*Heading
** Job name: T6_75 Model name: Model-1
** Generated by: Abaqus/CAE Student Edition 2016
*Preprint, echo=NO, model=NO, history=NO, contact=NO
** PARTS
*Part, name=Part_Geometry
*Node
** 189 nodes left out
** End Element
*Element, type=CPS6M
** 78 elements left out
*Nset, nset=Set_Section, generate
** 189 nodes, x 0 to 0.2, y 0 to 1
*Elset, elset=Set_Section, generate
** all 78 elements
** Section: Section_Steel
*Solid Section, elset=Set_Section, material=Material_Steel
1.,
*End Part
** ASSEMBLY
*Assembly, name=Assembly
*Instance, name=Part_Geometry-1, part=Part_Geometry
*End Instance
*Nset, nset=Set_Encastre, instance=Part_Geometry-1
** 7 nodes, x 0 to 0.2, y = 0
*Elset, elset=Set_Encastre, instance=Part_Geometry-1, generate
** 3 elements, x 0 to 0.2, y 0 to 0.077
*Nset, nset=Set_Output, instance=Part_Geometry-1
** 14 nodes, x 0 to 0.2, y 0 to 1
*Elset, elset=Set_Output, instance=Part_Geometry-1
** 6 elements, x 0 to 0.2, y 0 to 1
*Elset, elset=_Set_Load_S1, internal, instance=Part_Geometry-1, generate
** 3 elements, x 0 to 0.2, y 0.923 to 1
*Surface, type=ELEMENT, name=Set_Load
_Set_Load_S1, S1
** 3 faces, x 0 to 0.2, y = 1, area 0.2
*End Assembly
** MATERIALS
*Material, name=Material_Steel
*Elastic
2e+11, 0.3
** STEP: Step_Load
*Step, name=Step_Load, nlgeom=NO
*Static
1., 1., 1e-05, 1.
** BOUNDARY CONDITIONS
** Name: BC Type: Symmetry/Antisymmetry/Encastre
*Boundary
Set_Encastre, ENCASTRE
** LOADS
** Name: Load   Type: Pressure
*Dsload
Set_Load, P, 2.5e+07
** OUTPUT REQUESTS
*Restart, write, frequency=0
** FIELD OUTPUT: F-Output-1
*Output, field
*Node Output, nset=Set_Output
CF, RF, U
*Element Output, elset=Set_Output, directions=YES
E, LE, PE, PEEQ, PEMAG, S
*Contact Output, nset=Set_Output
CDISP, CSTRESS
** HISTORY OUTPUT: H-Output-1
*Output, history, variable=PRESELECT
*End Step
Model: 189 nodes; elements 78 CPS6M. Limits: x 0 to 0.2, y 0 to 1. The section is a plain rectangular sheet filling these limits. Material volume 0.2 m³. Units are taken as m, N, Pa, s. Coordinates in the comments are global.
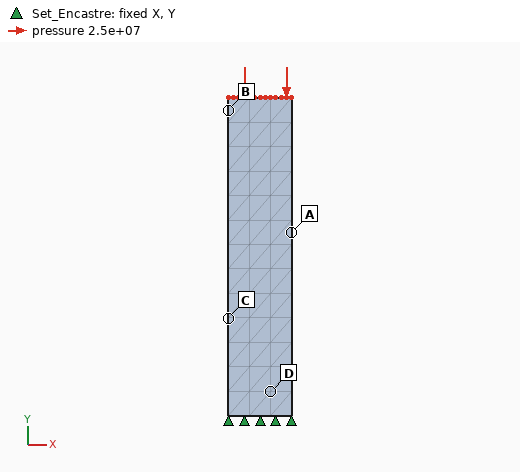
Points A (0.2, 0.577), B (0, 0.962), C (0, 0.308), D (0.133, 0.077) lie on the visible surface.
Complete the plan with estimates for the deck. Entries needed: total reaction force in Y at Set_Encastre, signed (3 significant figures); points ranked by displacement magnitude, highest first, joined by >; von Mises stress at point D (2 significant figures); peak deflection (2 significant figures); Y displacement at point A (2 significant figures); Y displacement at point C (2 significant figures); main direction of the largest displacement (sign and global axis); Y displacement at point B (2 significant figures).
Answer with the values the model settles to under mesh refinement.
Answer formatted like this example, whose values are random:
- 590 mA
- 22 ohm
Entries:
- 5.00e+06 N
- B > A > C > D
- 2.5e+07 Pa
- 1.2e-04 m
- -7.2e-05 m
- -3.8e-05 m
- -Y
- -1.2e-04 m
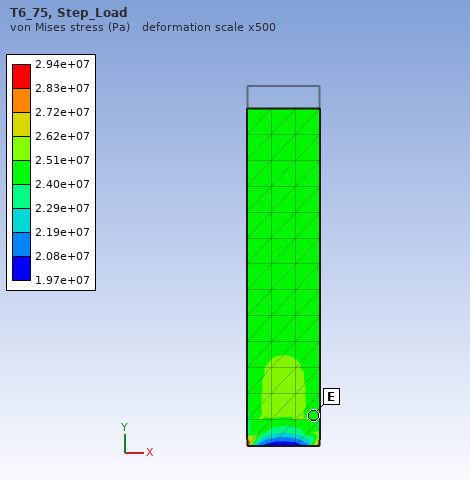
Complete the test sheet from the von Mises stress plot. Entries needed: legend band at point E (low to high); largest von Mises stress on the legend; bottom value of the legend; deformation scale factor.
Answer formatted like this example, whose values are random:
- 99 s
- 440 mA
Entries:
- 2.40e+07 to 2.51e+07 Pa
- 2.94e+07 Pa
- 1.97e+07 Pa
- 500
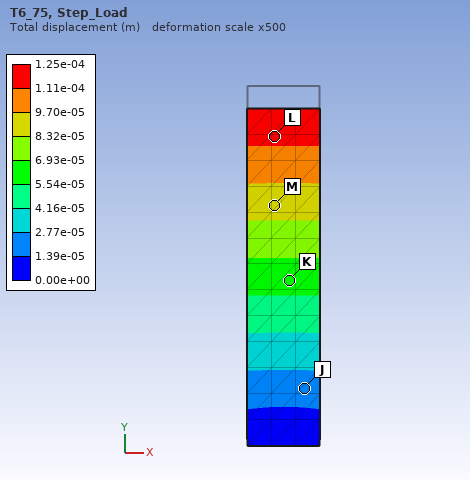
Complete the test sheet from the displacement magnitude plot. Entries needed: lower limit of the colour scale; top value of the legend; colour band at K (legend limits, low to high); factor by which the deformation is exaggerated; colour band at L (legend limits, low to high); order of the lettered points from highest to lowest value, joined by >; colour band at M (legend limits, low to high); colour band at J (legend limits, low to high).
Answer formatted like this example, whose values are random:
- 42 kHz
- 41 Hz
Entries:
- 0.00e+00 m
- 1.25e-04 m
- 5.54e-05 to 6.93e-05 m
- 500
- 1.11e-04 to 1.25e-04 m
- L > M > K > J
- 8.32e-05 to 9.70e-05 m
- 1.39e-05 to 2.77e-05 m
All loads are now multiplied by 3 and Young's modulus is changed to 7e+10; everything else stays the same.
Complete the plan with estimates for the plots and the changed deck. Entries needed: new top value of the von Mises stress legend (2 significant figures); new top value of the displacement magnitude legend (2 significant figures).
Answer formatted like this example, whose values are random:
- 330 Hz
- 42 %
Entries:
- 8.8e+07 Pa
- 0.0011 m
